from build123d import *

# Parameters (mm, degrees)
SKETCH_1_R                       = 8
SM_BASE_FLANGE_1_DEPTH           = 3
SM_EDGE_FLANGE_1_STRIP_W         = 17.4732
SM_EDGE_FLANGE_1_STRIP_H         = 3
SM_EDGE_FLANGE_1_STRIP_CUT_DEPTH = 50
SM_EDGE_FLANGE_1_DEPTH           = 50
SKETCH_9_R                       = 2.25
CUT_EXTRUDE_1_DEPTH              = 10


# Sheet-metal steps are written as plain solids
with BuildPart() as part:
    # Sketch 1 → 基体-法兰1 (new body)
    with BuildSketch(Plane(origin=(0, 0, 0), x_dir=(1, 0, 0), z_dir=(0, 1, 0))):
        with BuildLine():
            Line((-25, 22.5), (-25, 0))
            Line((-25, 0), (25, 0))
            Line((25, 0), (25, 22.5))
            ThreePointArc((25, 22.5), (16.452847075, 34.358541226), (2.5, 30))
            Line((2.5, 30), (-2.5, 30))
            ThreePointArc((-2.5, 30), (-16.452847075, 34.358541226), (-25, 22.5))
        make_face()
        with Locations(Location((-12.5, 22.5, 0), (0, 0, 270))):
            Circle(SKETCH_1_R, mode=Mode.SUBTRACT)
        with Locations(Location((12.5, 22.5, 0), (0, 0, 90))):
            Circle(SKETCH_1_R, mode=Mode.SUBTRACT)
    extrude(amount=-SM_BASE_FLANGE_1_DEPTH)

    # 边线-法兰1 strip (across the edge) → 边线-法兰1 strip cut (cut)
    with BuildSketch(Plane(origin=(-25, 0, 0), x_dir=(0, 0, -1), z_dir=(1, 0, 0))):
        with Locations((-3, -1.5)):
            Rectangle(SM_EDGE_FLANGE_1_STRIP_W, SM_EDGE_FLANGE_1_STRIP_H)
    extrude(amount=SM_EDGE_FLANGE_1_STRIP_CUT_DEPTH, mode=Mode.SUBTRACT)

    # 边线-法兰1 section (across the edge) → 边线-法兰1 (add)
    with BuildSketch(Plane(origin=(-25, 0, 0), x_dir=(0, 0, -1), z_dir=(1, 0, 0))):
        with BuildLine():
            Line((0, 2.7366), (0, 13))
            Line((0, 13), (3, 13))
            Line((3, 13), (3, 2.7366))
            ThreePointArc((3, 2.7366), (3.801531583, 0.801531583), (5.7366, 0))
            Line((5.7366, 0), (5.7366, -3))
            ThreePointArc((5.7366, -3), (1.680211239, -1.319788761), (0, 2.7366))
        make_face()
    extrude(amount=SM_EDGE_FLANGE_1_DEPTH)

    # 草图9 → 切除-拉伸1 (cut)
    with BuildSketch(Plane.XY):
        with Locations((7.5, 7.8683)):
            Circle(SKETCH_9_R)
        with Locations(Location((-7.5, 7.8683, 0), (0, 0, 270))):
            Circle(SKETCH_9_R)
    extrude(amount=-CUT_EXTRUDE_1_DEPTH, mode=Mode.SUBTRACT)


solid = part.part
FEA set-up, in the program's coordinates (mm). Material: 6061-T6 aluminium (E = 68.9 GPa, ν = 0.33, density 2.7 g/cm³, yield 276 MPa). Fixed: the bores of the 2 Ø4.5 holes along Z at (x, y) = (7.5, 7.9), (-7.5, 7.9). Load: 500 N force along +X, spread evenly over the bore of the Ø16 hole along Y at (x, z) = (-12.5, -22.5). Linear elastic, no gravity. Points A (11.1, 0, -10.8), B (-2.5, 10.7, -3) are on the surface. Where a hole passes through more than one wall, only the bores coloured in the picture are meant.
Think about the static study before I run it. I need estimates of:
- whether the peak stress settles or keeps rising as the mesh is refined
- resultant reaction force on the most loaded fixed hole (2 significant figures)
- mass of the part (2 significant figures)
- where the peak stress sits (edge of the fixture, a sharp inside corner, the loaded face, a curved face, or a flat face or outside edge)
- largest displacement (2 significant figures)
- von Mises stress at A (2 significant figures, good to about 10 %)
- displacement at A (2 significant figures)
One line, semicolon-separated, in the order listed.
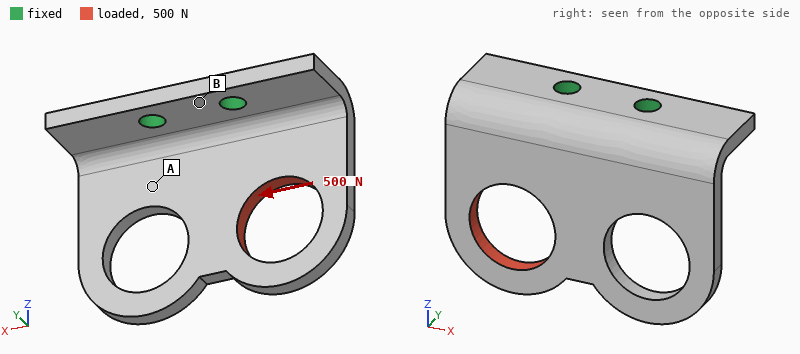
keeps rising; 630 N; 14 g; edge of the fixture; 0.13 mm; 34 MPa; 0.044 mm
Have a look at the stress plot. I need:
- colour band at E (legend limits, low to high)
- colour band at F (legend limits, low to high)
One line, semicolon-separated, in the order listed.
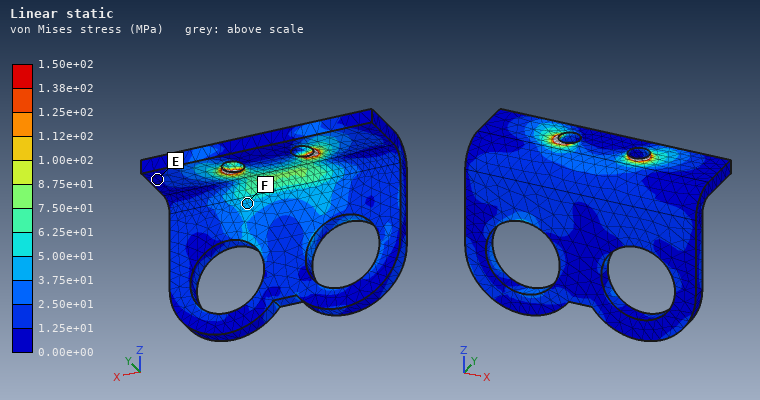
0.00e+00 to 1.25e+01 MPa; 3.75e+01 to 5.00e+01 MPa
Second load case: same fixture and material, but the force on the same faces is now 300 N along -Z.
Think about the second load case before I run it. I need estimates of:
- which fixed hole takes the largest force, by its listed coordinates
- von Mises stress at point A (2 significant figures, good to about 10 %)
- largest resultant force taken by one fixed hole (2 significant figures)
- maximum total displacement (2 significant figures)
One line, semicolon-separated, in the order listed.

(-7.5, 7.9); 11 MPa; 330 N; 97 µm
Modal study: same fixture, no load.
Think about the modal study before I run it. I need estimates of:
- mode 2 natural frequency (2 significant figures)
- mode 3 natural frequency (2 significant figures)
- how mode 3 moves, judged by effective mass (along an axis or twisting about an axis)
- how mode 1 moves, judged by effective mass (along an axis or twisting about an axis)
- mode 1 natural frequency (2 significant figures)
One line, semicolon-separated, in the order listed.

3400 Hz; 5200 Hz; along X; along Y; 2100 Hz
